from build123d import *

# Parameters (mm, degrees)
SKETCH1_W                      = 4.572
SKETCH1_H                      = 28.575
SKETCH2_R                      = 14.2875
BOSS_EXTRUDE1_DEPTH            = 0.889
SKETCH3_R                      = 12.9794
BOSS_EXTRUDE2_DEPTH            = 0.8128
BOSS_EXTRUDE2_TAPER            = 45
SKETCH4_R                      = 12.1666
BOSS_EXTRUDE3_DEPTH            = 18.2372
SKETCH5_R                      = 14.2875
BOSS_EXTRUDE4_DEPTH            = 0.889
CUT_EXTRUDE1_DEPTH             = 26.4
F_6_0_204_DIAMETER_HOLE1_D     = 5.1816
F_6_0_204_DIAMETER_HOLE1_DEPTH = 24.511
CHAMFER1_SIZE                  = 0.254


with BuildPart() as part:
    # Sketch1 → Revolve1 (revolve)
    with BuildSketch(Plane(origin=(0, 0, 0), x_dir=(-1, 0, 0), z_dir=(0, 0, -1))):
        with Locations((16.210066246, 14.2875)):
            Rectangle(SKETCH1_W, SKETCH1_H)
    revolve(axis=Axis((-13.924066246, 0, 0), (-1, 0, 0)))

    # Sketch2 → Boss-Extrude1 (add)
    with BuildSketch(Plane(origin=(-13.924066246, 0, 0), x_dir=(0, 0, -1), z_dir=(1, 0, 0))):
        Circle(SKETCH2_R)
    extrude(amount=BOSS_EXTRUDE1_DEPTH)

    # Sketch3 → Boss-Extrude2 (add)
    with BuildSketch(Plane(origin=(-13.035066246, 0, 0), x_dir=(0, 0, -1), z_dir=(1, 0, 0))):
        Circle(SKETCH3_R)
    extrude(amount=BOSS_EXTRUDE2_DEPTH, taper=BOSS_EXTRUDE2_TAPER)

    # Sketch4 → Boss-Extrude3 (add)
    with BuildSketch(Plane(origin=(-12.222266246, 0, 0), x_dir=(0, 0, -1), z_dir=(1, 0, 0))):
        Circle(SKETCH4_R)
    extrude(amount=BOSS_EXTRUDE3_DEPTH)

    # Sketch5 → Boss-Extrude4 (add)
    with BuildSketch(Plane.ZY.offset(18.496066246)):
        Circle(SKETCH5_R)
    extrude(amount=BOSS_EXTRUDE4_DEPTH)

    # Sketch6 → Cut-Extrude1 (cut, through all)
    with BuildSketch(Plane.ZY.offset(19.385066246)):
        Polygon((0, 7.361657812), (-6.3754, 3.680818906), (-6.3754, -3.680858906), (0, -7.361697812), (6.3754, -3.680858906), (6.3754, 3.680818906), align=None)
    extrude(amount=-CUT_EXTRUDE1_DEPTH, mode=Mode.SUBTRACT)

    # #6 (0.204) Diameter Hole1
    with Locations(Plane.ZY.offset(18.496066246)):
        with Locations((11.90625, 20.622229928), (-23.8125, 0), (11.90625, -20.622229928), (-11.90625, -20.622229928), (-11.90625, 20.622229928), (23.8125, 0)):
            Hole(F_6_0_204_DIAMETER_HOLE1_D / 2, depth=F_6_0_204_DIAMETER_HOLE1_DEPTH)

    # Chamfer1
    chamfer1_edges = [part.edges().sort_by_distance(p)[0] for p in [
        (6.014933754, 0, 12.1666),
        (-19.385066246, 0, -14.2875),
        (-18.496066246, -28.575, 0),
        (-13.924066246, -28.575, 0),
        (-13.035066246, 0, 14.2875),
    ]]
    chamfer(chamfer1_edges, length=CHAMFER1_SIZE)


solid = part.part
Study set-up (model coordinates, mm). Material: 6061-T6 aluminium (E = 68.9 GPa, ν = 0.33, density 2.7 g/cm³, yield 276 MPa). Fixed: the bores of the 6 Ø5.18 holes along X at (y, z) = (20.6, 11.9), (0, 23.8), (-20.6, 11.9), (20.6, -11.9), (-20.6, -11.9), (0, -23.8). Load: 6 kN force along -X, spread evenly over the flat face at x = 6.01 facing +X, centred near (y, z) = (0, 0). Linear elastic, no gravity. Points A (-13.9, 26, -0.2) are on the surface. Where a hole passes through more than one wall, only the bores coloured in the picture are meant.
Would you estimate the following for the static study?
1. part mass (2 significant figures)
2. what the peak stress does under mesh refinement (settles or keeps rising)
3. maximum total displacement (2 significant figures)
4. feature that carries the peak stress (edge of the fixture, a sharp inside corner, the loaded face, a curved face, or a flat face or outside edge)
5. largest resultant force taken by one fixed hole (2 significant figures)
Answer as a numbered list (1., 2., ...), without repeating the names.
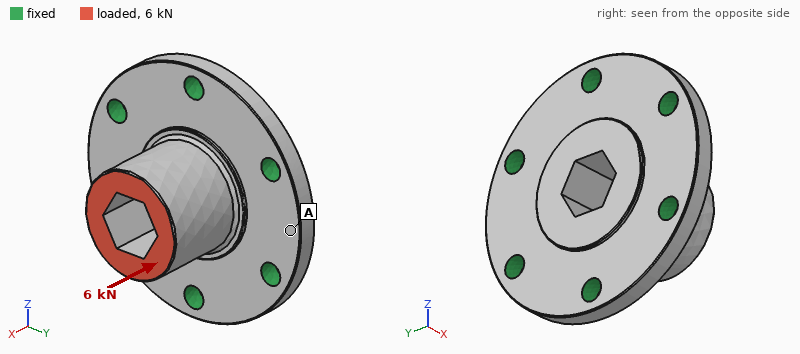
1. 47 g
2. keeps rising
3. 27 µm
4. edge of the fixture
5. 1.1 kN
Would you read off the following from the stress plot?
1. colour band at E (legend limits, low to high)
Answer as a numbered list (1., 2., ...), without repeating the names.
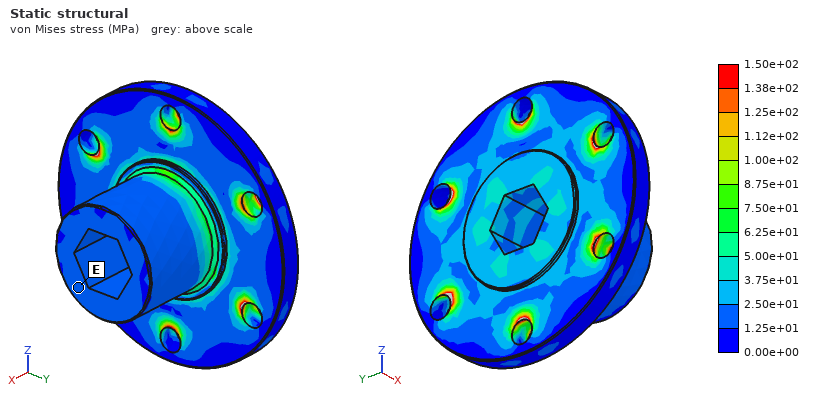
1. 1.25e+01 to 2.50e+01 MPa
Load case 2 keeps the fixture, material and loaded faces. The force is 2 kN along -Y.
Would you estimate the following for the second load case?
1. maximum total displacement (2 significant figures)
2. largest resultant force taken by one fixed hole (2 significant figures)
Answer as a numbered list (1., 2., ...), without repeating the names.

1. 37 µm
2. 810 N
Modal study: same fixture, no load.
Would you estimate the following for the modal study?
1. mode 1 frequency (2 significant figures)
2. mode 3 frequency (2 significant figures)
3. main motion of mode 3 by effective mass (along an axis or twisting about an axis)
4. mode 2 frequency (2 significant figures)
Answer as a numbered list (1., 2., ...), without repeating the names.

1. 14 kHz
2. 15 kHz
3. along X
4. 14 kHz
